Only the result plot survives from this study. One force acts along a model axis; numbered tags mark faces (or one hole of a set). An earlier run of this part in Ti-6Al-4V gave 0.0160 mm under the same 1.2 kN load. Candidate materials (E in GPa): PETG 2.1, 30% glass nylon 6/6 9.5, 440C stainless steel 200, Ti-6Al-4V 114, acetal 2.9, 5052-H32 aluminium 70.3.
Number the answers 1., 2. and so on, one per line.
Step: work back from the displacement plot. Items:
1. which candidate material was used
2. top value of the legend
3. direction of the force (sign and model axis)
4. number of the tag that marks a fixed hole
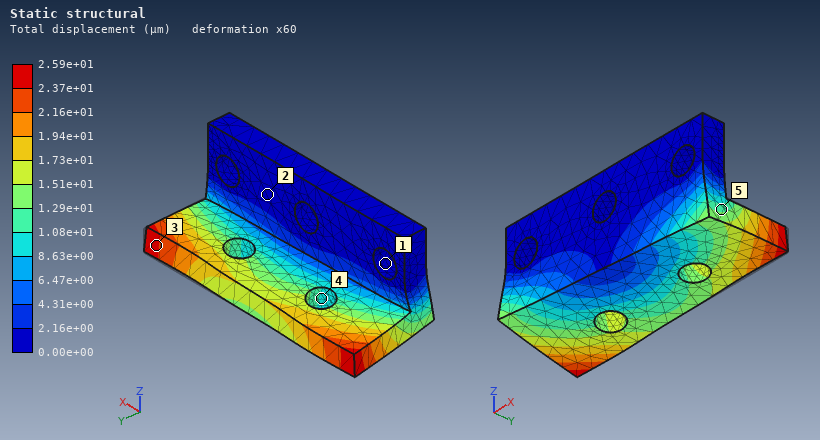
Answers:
1. 5052-H32 aluminium
2. 2.59e+01 µm
3. -X
4. 1
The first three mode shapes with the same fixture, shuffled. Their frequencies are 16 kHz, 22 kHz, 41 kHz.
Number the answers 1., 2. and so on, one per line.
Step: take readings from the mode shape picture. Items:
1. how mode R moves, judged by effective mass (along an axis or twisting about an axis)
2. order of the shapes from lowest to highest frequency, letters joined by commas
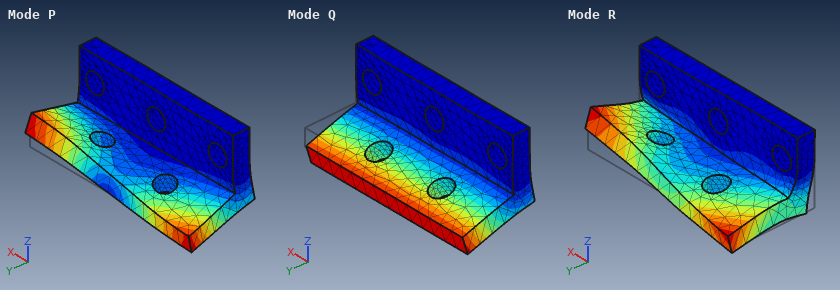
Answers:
1. along X
2. Q, P, R
